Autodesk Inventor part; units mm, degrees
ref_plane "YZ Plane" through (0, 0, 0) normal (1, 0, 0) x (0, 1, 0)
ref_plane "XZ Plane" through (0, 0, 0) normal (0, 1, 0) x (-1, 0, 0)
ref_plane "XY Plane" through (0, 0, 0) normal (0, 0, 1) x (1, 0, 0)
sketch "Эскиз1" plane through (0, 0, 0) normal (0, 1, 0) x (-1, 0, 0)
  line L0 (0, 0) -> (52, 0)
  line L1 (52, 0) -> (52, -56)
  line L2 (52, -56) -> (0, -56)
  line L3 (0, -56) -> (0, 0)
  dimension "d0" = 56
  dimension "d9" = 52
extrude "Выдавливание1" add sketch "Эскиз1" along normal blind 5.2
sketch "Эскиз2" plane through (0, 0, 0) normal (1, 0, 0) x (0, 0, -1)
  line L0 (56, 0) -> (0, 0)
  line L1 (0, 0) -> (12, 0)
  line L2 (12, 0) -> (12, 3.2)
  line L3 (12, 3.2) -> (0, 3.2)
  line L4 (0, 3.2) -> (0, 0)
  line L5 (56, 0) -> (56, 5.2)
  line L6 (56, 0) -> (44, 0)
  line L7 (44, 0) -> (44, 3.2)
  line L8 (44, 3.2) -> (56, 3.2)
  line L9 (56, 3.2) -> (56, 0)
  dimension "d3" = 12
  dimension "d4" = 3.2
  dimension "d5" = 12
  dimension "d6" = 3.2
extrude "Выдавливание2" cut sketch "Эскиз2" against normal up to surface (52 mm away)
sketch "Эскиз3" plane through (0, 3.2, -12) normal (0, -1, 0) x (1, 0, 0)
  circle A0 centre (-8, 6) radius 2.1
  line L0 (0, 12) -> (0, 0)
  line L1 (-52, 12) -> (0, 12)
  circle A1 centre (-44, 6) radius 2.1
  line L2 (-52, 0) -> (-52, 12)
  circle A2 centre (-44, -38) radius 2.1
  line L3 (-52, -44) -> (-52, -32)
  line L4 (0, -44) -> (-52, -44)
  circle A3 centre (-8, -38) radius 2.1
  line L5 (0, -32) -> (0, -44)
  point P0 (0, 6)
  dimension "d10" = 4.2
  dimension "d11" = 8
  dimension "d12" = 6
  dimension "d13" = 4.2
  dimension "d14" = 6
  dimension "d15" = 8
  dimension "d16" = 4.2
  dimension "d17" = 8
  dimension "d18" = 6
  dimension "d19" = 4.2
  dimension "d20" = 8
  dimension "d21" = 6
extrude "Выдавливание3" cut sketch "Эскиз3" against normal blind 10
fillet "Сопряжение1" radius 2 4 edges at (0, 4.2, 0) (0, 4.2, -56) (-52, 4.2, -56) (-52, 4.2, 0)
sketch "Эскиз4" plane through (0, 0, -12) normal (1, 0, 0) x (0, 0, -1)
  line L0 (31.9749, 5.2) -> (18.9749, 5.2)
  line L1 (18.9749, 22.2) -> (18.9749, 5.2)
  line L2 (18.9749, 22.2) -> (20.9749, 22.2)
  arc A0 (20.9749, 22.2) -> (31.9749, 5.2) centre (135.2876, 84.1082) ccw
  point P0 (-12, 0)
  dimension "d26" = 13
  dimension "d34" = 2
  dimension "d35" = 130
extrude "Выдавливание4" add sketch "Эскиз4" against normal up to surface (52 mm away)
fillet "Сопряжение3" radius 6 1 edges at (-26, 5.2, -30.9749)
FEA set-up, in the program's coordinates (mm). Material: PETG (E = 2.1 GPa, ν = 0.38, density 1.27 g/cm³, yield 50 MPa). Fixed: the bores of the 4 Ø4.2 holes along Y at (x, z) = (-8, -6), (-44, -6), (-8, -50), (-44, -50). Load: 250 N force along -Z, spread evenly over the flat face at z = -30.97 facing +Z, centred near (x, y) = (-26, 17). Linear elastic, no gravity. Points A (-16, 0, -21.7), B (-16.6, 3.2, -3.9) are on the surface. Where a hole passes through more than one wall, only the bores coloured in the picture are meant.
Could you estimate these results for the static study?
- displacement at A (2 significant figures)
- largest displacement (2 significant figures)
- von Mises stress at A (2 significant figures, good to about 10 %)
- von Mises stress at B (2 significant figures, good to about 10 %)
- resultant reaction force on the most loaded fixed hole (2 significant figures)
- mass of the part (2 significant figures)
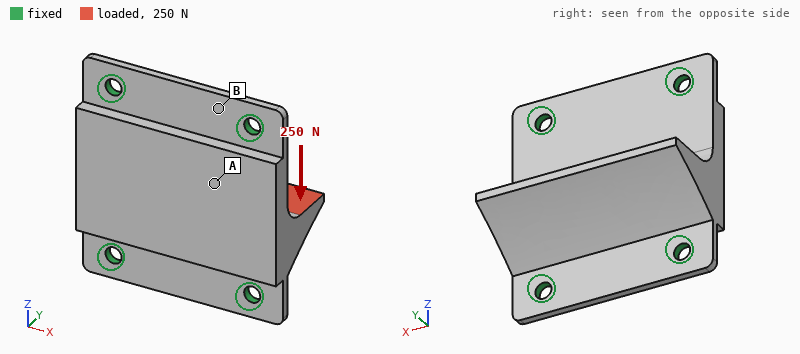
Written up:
0.10 mm
0.21 mm
3.6 MPa
1.5 MPa
130 N
23 g
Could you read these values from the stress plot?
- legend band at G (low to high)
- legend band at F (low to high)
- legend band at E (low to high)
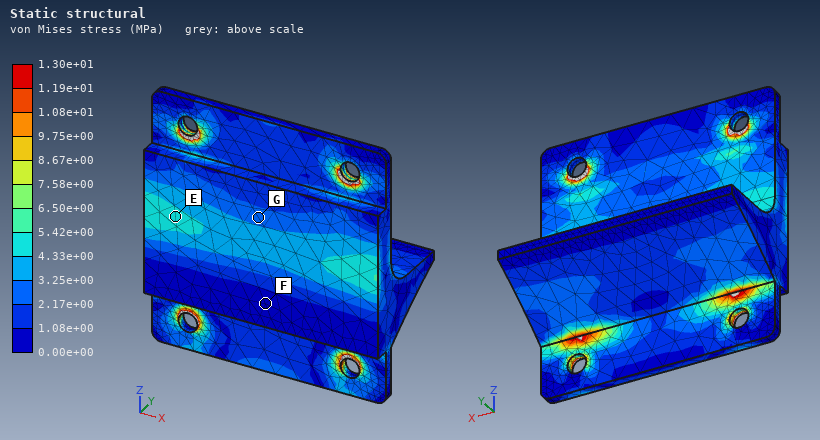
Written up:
2.17e+00 to 3.25e+00 MPa
0.00e+00 to 1.08e+00 MPa
4.33e+00 to 5.42e+00 MPa
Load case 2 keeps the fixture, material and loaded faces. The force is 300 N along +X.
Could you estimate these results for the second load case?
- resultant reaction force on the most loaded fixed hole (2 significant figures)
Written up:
130 N
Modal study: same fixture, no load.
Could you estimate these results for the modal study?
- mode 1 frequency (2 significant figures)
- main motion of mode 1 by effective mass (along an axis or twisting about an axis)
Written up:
1500 Hz
along Y
